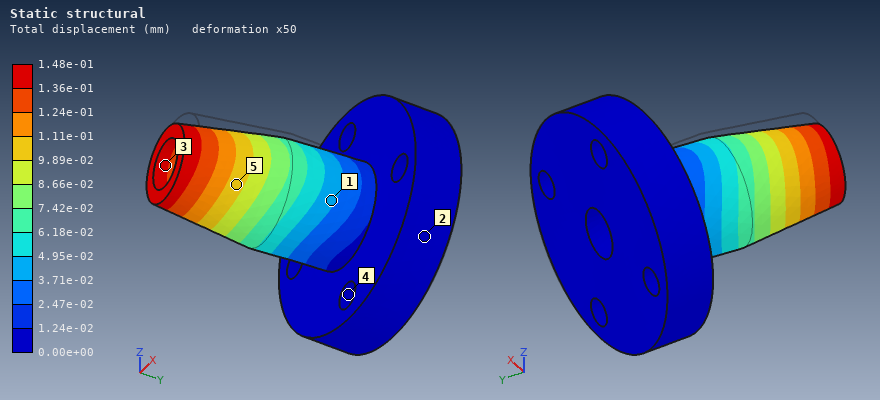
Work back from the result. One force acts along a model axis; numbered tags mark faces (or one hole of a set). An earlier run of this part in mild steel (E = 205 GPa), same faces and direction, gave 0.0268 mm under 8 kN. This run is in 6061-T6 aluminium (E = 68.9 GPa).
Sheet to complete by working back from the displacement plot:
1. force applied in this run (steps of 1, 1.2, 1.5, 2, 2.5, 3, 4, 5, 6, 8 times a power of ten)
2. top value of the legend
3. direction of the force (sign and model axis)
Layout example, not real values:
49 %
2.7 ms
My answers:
15 kN
1.48e-01 mm
-X
